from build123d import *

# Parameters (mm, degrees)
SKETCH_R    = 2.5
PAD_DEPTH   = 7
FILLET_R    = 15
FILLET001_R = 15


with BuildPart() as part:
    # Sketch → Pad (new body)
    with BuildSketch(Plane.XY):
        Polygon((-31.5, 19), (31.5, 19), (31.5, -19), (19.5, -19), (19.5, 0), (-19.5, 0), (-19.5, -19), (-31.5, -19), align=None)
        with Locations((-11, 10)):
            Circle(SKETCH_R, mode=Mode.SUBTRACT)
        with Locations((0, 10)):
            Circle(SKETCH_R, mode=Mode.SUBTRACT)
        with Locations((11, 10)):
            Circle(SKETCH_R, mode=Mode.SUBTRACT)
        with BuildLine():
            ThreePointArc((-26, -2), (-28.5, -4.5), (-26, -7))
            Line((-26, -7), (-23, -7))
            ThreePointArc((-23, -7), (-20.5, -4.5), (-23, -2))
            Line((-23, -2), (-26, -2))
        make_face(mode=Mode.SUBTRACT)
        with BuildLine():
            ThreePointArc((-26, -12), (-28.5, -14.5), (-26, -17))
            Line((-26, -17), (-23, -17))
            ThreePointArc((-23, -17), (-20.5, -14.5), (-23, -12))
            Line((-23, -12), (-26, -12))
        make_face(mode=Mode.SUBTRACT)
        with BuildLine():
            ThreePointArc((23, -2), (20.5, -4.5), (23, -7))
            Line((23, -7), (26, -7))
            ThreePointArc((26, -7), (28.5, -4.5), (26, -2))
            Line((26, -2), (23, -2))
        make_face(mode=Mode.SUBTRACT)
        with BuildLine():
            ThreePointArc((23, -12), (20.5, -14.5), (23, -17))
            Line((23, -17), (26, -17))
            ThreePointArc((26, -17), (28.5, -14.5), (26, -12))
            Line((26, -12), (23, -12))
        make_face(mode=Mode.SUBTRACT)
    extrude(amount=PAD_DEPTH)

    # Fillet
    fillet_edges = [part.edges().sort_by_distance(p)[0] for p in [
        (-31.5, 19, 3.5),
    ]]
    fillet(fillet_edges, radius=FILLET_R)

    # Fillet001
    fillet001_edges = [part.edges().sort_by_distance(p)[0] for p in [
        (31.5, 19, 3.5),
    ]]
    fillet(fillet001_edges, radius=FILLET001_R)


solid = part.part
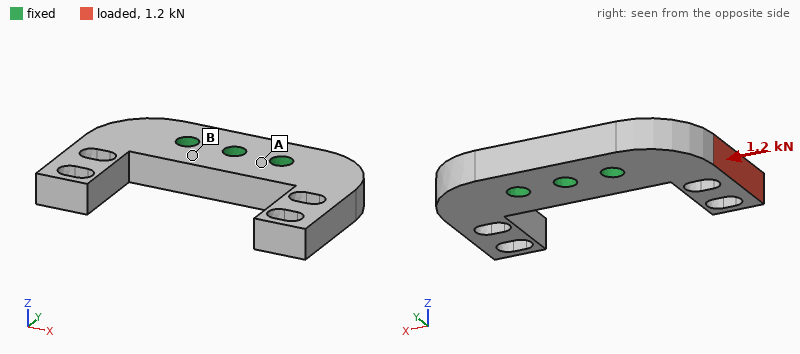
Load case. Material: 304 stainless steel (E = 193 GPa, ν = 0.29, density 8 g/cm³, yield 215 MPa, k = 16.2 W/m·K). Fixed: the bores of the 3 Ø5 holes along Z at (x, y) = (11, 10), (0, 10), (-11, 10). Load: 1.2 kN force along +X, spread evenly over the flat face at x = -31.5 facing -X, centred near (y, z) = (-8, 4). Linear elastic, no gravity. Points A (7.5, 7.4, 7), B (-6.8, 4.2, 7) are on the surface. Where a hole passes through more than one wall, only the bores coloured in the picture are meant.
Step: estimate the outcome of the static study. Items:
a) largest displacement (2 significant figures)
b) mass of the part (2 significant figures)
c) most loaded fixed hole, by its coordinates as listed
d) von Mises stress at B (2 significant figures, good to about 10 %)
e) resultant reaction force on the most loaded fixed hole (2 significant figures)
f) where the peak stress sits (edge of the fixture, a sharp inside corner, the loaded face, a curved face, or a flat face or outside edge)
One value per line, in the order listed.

43 µm
76 g
(-11, 10)
26 MPa
1.2 kN
a curved face
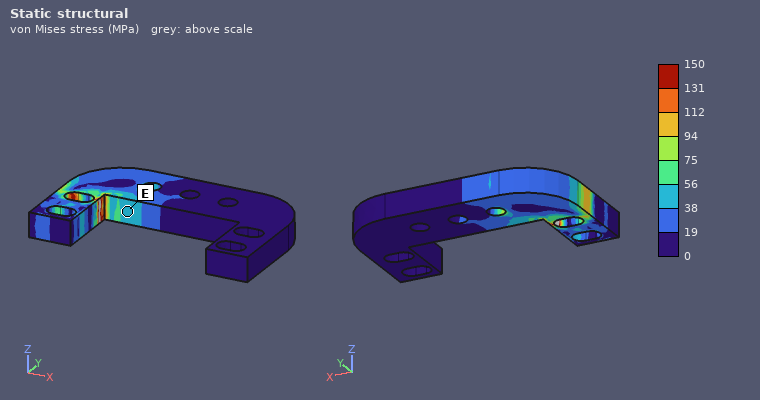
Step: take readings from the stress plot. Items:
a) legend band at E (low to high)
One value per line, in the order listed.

38 to 56 MPa
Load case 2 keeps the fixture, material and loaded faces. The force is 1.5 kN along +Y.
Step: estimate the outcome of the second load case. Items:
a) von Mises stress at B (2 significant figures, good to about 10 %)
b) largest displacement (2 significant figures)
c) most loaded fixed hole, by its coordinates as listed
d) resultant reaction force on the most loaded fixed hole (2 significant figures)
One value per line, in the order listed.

31 MPa
40 µm
(-11, 10)
2.7 kN
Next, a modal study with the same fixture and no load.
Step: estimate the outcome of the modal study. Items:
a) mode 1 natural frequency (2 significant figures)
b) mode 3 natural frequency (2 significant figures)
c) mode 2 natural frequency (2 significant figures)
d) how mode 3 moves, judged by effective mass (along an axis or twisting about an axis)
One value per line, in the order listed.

5600 Hz
9200 Hz
5600 Hz
along X
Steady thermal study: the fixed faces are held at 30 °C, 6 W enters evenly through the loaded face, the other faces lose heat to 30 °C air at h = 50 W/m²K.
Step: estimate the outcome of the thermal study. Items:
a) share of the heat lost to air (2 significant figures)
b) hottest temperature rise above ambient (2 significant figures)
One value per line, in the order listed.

50 %
78 K
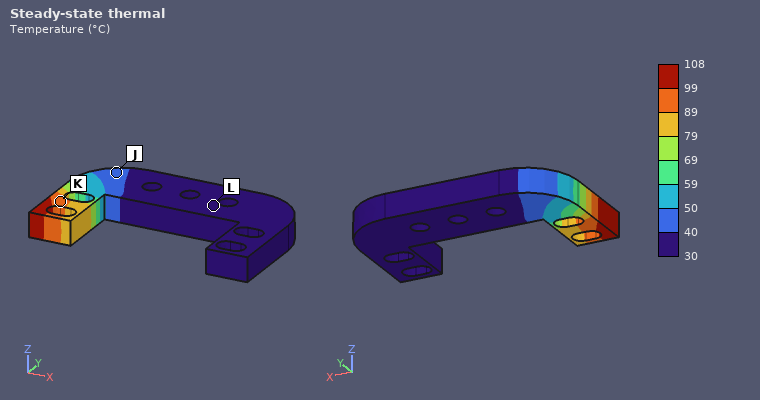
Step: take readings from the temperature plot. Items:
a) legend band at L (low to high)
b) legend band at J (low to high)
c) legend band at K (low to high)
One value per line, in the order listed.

30 to 40 °C
40 to 50 °C
89 to 99 °C
